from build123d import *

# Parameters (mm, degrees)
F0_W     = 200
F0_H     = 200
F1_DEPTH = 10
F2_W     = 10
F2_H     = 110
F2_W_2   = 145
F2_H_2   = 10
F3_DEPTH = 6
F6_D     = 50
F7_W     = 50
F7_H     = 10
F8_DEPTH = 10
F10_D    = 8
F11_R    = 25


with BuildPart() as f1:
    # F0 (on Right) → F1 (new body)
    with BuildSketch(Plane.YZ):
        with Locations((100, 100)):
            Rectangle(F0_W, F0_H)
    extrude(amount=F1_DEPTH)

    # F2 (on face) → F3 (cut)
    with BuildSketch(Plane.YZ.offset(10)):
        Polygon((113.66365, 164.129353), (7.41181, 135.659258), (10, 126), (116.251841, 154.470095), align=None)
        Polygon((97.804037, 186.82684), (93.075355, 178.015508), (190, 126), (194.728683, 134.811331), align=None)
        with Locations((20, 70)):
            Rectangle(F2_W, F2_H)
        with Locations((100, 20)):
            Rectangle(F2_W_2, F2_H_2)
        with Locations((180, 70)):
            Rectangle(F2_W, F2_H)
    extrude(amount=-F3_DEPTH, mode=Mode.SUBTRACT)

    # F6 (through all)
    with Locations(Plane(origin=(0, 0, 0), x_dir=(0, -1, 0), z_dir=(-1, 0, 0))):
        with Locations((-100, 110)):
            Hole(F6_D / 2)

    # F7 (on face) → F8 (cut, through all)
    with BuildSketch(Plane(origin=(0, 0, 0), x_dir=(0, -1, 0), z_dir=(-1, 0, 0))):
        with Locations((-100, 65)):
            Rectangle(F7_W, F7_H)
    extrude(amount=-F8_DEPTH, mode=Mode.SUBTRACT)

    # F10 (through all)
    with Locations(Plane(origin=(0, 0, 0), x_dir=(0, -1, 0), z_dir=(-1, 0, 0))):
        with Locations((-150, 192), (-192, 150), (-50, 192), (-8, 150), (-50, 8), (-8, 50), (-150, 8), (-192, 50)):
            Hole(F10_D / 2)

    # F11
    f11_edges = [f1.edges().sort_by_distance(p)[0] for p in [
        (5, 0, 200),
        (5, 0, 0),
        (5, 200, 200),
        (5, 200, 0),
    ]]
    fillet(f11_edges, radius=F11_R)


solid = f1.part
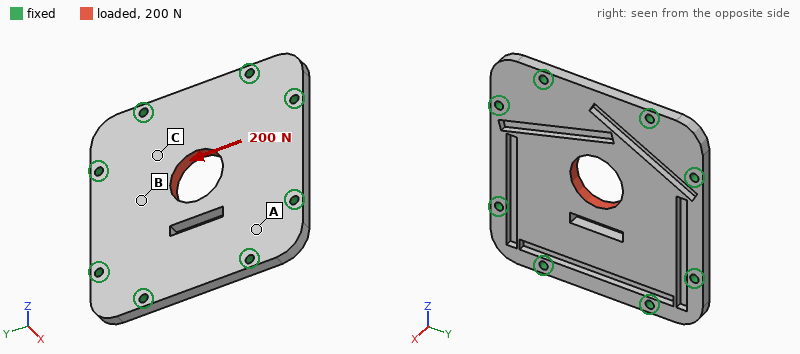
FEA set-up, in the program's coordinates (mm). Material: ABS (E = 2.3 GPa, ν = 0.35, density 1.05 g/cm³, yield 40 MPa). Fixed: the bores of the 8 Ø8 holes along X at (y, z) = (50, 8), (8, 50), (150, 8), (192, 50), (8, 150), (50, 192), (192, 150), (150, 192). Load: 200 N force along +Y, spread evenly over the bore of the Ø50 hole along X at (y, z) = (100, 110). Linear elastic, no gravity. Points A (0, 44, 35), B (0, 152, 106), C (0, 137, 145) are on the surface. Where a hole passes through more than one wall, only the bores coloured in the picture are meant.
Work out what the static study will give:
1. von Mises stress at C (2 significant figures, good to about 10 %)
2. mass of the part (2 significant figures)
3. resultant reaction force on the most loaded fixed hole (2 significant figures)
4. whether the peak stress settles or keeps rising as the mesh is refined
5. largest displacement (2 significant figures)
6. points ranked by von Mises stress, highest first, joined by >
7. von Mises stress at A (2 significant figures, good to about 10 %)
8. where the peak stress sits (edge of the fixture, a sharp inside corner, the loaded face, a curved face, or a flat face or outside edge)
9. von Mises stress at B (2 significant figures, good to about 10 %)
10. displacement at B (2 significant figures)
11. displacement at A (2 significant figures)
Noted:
0.15 MPa
350 g
41 N
keeps rising
7.0 µm
C > B > A
0.037 MPa
edge of the fixture
0.093 MPa
5.1 µm
1.3 µm
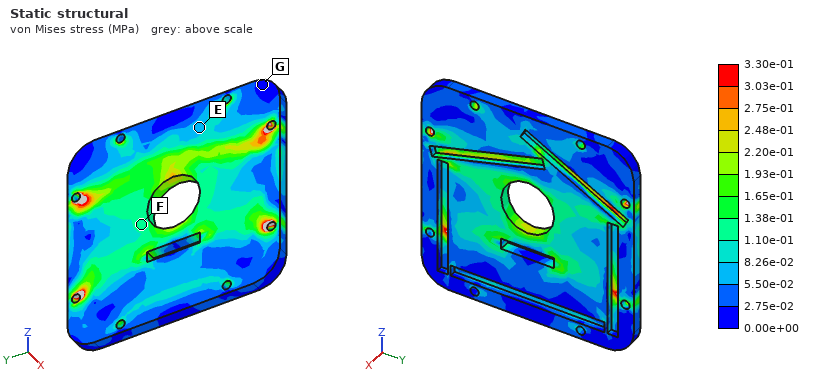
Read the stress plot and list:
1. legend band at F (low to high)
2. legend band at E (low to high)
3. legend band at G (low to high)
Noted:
1.10e-01 to 1.38e-01 MPa
5.50e-02 to 8.26e-02 MPa
0.00e+00 to 2.75e-02 MPa
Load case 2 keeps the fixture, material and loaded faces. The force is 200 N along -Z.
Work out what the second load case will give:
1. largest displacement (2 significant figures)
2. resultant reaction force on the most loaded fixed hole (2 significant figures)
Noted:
11 µm
40 N
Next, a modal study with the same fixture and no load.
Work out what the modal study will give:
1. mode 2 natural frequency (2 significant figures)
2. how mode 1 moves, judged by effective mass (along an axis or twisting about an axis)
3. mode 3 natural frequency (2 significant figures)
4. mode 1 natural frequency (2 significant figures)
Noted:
940 Hz
along X
940 Hz
480 Hz
